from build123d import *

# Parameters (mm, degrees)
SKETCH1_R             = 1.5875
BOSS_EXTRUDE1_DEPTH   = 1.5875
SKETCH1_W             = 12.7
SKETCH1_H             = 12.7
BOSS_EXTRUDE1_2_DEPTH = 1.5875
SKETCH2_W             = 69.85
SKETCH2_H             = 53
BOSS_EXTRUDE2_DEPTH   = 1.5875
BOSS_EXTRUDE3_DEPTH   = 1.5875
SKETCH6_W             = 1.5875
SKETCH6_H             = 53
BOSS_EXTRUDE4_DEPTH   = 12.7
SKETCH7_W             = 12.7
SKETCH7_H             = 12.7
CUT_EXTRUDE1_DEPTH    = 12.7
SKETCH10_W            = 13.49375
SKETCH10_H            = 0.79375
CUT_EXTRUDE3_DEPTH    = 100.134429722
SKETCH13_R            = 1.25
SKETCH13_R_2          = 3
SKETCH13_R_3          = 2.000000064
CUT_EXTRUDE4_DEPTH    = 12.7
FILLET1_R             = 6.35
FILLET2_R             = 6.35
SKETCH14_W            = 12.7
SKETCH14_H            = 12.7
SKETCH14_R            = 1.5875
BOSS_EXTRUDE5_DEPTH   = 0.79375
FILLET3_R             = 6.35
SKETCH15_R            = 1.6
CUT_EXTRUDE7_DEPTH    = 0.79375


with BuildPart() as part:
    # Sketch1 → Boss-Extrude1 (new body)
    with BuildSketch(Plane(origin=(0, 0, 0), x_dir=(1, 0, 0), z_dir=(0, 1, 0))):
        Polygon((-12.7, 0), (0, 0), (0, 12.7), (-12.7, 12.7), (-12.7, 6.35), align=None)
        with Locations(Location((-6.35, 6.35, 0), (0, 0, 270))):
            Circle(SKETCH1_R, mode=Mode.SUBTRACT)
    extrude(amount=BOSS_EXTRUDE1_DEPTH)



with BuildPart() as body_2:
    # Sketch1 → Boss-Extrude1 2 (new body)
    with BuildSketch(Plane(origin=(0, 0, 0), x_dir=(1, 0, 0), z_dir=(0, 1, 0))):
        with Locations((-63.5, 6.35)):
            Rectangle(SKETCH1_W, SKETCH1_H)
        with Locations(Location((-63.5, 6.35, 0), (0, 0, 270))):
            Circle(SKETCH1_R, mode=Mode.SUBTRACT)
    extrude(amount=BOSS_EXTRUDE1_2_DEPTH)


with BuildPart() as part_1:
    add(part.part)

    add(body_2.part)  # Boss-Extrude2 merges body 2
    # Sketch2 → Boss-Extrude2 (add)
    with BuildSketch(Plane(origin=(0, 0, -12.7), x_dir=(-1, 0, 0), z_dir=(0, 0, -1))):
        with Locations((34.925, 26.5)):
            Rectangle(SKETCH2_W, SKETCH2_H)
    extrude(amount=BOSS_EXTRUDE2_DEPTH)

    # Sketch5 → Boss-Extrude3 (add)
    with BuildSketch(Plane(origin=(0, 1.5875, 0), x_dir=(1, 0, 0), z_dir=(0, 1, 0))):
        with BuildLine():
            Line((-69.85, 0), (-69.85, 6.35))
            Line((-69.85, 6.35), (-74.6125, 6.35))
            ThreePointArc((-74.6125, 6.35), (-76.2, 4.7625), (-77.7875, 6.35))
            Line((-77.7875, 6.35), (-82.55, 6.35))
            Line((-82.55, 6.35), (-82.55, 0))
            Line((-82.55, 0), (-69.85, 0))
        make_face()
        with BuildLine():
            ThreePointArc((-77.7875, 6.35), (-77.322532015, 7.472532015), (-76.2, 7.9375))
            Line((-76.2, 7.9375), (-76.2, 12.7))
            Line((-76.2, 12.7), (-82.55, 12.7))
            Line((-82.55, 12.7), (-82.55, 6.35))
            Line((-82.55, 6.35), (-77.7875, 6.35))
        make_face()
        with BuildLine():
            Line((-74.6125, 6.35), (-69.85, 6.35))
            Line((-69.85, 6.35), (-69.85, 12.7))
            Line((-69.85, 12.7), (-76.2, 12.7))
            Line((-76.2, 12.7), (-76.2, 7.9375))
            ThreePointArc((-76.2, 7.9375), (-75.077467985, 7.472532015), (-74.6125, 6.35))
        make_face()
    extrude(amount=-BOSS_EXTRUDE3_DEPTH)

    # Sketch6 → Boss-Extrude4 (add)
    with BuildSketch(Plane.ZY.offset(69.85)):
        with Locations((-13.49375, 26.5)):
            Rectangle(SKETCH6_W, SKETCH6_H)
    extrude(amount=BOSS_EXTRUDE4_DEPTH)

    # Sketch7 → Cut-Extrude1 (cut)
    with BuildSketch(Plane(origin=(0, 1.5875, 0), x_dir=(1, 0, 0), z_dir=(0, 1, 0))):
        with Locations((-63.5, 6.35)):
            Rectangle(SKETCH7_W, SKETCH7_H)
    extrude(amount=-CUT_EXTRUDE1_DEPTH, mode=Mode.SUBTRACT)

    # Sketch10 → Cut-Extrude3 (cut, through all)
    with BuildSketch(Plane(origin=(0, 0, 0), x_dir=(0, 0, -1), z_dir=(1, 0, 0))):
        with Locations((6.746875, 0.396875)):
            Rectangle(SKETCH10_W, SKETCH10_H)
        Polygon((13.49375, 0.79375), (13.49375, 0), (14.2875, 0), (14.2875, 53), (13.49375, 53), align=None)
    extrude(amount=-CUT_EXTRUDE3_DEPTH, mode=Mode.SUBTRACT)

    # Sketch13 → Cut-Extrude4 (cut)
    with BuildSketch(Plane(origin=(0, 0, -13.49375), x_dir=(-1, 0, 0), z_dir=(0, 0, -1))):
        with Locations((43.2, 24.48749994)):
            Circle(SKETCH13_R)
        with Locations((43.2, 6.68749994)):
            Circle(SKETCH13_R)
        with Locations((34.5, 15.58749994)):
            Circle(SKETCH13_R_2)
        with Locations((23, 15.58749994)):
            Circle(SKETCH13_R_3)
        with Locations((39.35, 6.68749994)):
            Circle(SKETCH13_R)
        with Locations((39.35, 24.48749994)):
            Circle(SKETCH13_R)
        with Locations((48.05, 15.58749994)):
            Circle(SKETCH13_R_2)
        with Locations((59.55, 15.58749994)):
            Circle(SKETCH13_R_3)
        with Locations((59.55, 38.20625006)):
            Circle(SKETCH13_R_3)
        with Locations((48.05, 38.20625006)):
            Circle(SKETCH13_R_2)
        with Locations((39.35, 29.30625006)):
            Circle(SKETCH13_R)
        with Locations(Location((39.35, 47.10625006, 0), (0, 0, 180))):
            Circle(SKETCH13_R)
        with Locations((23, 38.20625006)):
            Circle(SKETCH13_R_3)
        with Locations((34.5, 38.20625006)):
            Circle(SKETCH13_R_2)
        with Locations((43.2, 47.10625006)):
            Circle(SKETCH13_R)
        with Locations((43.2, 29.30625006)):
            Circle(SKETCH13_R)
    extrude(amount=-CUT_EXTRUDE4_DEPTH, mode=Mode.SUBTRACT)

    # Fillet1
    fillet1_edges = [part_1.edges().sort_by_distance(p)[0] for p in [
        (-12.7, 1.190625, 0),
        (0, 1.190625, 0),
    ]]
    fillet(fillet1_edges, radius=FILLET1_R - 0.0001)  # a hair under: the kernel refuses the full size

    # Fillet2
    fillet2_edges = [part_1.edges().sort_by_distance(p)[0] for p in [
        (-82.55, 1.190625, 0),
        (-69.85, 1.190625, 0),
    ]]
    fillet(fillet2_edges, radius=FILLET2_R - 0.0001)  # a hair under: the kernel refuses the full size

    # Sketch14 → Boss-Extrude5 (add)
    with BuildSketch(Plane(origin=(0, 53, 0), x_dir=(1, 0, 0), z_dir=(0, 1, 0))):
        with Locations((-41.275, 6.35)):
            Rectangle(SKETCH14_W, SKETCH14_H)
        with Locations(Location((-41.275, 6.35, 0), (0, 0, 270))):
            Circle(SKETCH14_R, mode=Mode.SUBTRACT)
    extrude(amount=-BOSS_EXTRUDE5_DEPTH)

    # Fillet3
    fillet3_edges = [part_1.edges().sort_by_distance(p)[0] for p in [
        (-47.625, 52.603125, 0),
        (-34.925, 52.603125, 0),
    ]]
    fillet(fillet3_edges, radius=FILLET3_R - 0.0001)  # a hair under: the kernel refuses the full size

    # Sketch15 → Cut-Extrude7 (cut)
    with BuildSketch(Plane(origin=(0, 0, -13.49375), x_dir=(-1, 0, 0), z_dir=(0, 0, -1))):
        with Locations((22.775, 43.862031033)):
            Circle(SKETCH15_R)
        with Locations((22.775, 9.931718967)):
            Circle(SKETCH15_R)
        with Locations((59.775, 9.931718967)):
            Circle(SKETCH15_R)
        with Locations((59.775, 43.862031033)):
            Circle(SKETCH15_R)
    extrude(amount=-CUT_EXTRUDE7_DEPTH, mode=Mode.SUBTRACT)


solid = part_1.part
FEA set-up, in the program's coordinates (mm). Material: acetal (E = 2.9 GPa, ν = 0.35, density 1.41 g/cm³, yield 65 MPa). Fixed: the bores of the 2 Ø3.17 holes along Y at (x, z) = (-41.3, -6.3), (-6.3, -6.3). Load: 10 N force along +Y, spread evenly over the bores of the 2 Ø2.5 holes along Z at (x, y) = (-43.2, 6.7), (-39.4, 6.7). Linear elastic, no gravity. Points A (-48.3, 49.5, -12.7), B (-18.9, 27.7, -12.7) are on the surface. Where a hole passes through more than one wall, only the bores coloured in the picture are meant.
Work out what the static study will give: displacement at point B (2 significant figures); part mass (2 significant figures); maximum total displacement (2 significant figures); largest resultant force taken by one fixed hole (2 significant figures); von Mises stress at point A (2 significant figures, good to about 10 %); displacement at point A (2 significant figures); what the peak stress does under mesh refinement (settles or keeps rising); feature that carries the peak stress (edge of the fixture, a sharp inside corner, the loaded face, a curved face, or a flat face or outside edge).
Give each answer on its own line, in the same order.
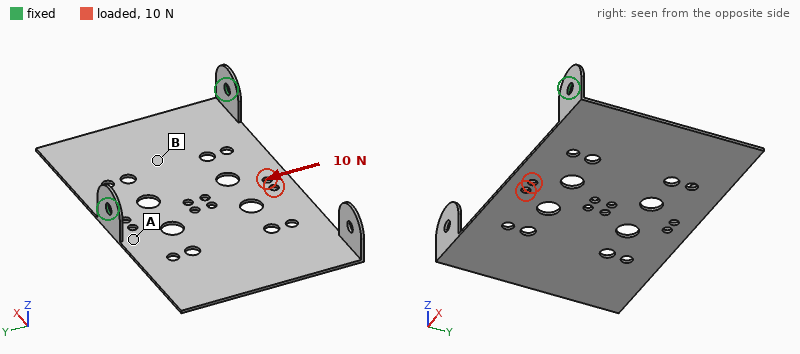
0.18 mm
5.0 g
1.2 mm
6.2 N
2.4 MPa
0.19 mm
keeps rising
edge of the fixture
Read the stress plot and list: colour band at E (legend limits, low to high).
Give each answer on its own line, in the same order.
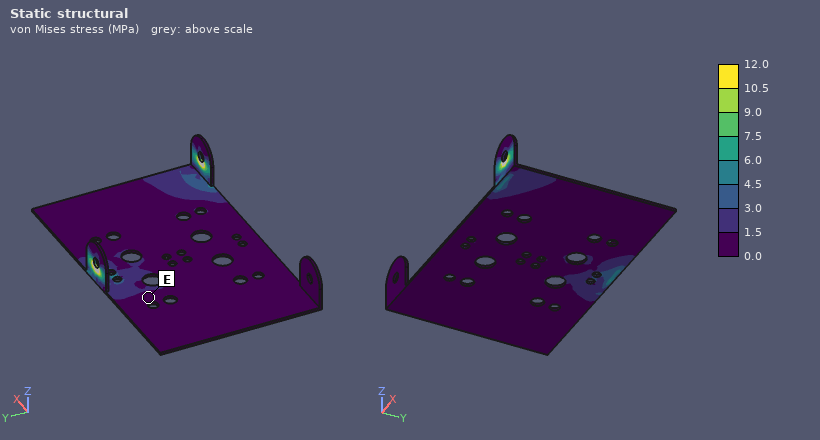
0.0 to 1.5 MPa
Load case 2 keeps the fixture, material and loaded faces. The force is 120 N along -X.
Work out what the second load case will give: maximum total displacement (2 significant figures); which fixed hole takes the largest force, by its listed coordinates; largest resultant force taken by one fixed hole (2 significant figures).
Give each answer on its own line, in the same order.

1.0 mm
(-6.3, -6.3)
110 N
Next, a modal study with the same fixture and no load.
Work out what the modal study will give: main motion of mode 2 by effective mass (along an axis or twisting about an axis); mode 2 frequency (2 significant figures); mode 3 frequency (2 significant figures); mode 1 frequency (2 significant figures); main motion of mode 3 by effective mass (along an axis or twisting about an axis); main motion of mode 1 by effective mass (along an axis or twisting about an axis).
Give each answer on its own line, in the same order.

twisting about X
160 Hz
170 Hz
48 Hz
along Z
along Z
